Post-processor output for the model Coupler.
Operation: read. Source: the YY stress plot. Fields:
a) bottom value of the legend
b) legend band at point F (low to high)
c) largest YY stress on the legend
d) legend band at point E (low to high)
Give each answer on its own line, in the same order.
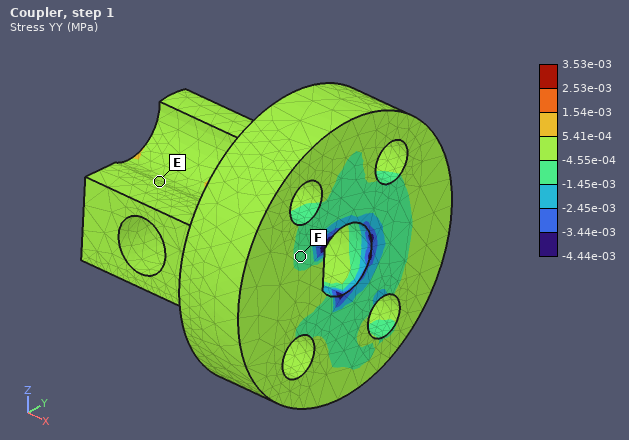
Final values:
-4.44e-03 MPa
-1.45e-03 to -4.55e-04 MPa
3.53e-03 MPa
-4.55e-04 to 5.41e-04 MPa
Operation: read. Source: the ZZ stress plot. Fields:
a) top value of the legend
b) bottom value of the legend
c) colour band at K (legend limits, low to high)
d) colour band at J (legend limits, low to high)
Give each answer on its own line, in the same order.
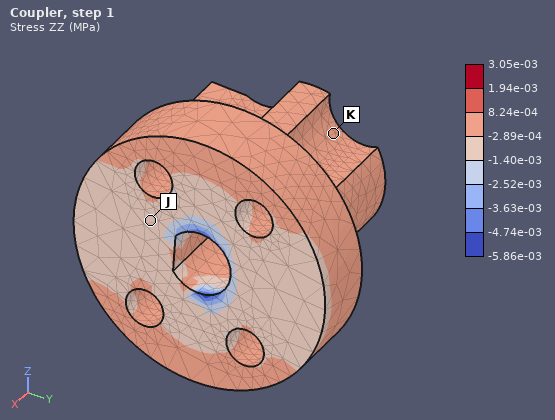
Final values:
3.05e-03 MPa
-5.86e-03 MPa
-2.89e-04 to 8.24e-04 MPa
-1.40e-03 to -2.89e-04 MPa
